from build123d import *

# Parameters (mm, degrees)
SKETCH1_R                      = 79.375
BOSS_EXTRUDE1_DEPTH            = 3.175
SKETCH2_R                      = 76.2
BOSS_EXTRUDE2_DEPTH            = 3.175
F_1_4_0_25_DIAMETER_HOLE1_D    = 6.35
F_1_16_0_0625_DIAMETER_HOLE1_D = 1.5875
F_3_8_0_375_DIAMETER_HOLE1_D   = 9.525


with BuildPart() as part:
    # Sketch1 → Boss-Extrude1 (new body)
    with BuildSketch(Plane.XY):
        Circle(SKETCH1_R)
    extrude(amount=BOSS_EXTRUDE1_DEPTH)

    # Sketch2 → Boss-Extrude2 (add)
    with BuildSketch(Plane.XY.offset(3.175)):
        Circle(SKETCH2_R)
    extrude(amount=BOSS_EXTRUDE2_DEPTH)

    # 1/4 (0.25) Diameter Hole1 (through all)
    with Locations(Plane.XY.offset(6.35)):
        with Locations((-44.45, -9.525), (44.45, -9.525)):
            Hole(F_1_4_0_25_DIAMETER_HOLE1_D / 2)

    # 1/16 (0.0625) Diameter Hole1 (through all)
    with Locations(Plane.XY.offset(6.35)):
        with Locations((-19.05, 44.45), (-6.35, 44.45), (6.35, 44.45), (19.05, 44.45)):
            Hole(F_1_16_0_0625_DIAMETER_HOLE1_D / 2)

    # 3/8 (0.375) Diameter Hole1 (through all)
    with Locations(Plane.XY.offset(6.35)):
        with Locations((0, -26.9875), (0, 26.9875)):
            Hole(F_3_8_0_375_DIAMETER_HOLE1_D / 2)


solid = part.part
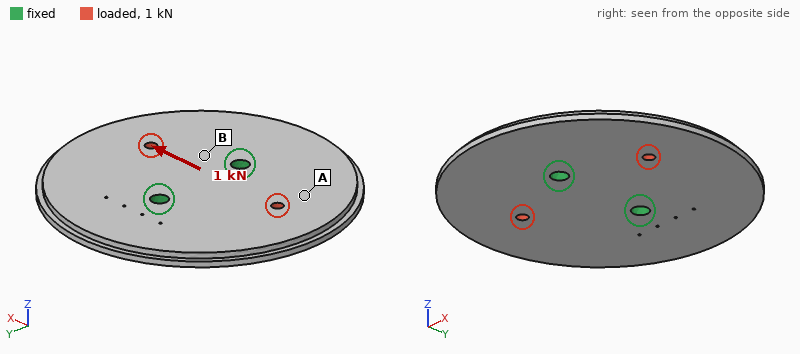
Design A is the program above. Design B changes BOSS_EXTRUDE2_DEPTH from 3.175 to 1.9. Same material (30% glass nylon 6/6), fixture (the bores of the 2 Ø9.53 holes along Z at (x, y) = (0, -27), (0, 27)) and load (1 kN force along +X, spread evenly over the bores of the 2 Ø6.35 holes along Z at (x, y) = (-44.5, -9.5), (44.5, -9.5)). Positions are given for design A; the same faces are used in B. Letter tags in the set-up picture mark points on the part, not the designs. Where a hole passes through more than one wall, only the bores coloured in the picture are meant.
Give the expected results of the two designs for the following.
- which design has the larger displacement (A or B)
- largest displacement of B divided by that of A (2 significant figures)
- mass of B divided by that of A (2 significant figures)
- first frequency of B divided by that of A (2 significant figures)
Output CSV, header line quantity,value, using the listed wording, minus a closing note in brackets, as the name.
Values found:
quantity,value
which design has the larger displacement,B
largest displacement of B divided by that of A,1.2
mass of B divided by that of A,0.81
first frequency of B divided by that of A,0.81
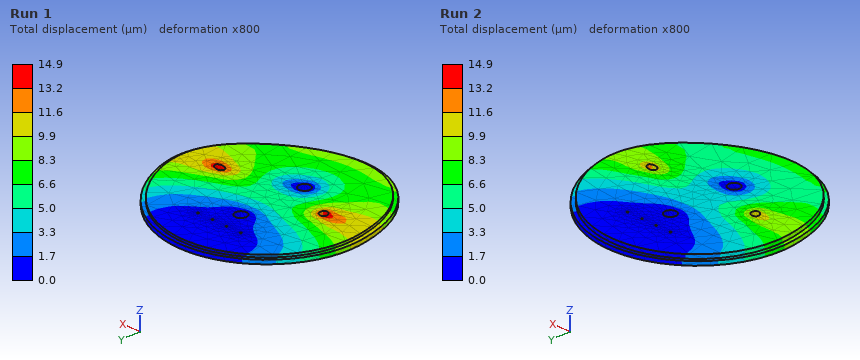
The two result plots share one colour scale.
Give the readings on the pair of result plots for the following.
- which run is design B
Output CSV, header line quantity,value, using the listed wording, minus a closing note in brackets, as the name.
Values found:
quantity,value
which run is design B,Run 1
